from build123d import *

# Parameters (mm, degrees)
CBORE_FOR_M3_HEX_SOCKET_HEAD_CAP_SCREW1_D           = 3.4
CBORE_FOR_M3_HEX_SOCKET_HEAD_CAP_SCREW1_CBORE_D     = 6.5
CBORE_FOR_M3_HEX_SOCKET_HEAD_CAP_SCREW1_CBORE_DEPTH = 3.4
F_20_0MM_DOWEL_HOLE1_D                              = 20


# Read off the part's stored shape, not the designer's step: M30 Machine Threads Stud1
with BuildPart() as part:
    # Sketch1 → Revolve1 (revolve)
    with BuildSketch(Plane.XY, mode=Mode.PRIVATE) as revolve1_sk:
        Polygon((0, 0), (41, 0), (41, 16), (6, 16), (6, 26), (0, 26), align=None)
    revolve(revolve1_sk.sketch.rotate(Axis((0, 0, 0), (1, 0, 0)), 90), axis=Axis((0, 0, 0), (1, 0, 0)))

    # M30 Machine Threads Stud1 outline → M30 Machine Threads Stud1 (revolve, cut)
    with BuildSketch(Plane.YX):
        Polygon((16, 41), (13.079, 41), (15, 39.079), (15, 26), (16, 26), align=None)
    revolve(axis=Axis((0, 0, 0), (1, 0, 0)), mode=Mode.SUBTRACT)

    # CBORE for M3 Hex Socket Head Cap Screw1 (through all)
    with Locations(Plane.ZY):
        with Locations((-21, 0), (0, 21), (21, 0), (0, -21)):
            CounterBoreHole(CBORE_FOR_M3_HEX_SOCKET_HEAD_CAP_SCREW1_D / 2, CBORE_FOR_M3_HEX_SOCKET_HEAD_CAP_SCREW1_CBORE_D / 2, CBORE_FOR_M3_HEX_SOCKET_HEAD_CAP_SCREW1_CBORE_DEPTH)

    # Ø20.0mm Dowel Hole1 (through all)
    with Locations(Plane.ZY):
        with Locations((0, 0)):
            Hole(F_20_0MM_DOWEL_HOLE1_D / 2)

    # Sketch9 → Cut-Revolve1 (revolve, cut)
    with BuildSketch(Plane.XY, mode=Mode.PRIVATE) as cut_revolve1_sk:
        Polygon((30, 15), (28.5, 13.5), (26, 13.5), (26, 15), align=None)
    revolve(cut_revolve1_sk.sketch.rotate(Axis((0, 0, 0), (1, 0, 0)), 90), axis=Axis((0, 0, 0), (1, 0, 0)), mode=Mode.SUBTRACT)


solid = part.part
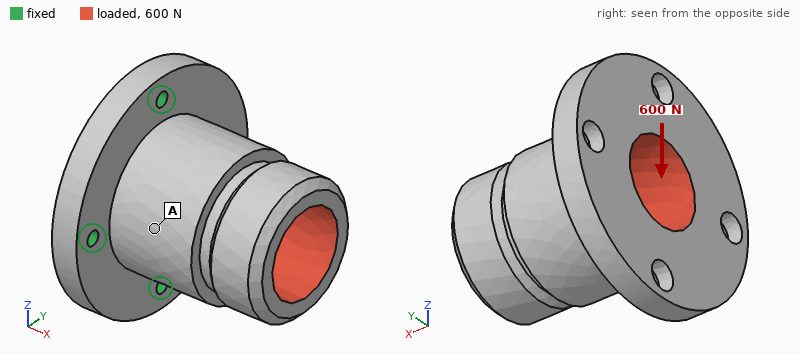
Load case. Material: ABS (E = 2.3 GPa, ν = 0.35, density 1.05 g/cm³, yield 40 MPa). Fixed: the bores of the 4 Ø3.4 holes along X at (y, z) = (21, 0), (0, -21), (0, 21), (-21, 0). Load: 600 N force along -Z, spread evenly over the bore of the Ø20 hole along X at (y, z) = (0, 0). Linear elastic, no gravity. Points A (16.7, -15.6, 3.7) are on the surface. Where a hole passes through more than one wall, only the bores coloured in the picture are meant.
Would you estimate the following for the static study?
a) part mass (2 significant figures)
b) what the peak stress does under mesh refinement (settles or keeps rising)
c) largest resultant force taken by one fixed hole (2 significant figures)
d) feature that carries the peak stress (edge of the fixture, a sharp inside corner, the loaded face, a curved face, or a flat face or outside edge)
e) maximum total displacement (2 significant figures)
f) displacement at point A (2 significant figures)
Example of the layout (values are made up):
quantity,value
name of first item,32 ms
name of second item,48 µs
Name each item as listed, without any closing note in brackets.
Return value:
quantity,value
part mass,27 g
what the peak stress does under mesh refinement,keeps rising
largest resultant force taken by one fixed hole,270 N
feature that carries the peak stress,edge of the fixture
maximum total displacement,0.23 mm
displacement at point A,0.081 mm
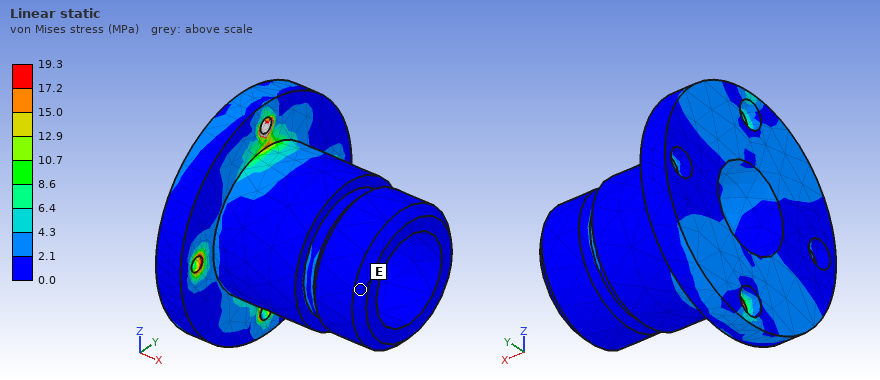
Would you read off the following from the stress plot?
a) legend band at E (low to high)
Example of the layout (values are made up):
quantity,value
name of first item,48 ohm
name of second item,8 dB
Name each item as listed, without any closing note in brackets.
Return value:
quantity,value
legend band at E,0.0 to 2.1 MPa
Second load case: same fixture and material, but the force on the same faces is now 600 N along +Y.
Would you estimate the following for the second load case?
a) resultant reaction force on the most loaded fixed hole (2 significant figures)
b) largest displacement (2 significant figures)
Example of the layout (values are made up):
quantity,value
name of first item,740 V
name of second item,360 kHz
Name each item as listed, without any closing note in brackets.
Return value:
quantity,value
resultant reaction force on the most loaded fixed hole,270 N
largest displacement,0.23 mm
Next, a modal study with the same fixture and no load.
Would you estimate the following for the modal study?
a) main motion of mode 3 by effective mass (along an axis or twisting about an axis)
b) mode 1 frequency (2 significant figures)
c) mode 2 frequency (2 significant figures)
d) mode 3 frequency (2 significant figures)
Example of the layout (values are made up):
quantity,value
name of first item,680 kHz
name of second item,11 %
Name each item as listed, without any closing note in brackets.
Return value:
quantity,value
main motion of mode 3 by effective mass,along X
mode 1 frequency,2300 Hz
mode 2 frequency,2300 Hz
mode 3 frequency,3700 Hz
